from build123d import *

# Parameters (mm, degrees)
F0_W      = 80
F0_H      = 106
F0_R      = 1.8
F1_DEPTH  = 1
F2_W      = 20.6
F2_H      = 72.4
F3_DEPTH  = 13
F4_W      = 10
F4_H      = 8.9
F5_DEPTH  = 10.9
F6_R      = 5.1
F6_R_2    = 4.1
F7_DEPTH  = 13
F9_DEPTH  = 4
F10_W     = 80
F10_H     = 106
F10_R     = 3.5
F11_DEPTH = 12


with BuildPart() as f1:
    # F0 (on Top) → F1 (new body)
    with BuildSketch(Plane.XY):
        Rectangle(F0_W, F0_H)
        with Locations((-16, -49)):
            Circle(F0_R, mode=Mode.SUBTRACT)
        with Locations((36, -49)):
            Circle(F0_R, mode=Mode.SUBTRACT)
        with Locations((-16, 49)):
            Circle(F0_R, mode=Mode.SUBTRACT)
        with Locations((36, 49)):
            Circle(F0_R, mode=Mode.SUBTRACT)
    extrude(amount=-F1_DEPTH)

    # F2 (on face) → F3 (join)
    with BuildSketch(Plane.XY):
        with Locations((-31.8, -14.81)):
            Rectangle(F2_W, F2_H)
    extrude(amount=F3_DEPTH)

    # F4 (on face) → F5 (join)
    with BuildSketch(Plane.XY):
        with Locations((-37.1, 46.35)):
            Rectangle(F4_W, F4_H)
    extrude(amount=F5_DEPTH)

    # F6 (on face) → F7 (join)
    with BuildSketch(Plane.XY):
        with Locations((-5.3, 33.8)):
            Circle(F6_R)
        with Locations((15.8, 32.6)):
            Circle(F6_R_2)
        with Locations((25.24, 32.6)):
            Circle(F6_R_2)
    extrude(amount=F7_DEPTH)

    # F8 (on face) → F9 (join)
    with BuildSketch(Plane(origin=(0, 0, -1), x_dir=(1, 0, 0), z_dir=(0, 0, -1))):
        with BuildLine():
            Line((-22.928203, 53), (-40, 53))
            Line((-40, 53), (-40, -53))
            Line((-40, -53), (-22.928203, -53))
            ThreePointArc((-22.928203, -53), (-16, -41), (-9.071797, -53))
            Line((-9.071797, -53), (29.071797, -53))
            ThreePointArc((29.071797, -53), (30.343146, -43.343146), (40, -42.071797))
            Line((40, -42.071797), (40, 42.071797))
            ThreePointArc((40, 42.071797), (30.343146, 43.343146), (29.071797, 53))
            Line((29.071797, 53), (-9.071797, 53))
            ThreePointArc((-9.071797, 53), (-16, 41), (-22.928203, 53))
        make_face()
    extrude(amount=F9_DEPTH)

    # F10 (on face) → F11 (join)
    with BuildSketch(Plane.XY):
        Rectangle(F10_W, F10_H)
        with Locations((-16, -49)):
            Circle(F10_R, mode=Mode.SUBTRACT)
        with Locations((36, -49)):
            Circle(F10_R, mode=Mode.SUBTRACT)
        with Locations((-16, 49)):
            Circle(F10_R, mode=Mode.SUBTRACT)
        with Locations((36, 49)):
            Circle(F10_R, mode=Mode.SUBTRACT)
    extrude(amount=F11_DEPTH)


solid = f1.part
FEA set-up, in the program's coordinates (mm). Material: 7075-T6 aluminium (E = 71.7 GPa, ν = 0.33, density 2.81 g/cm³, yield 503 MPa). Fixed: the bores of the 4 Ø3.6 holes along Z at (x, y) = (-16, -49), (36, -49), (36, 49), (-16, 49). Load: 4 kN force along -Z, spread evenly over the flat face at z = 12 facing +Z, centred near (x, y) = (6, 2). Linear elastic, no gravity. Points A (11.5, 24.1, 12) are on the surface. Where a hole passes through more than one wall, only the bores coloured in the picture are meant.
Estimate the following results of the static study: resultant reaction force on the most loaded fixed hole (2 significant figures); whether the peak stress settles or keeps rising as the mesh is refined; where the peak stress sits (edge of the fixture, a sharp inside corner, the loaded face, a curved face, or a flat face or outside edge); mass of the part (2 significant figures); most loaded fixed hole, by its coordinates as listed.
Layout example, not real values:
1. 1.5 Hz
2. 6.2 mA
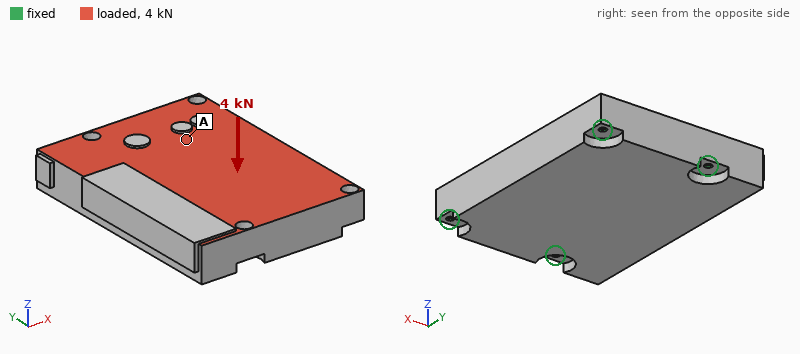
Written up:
1. 1.3 kN
2. keeps rising
3. edge of the fixture
4. 400 g
5. (-16, 49)
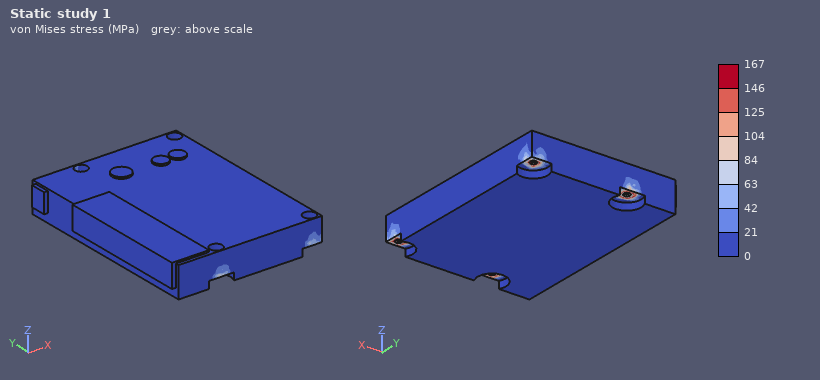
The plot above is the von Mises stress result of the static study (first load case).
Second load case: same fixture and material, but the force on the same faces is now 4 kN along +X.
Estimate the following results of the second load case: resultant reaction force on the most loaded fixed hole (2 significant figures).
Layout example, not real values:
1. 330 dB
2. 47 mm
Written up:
1. 1.3 kN
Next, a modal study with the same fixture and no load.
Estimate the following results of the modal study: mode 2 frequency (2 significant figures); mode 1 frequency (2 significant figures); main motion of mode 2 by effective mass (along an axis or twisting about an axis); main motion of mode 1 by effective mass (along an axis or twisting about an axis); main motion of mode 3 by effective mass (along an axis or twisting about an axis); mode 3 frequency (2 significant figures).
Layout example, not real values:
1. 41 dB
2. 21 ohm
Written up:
1. 3900 Hz
2. 2800 Hz
3. along Z
4. along Z
5. along Y
6. 5800 Hz
